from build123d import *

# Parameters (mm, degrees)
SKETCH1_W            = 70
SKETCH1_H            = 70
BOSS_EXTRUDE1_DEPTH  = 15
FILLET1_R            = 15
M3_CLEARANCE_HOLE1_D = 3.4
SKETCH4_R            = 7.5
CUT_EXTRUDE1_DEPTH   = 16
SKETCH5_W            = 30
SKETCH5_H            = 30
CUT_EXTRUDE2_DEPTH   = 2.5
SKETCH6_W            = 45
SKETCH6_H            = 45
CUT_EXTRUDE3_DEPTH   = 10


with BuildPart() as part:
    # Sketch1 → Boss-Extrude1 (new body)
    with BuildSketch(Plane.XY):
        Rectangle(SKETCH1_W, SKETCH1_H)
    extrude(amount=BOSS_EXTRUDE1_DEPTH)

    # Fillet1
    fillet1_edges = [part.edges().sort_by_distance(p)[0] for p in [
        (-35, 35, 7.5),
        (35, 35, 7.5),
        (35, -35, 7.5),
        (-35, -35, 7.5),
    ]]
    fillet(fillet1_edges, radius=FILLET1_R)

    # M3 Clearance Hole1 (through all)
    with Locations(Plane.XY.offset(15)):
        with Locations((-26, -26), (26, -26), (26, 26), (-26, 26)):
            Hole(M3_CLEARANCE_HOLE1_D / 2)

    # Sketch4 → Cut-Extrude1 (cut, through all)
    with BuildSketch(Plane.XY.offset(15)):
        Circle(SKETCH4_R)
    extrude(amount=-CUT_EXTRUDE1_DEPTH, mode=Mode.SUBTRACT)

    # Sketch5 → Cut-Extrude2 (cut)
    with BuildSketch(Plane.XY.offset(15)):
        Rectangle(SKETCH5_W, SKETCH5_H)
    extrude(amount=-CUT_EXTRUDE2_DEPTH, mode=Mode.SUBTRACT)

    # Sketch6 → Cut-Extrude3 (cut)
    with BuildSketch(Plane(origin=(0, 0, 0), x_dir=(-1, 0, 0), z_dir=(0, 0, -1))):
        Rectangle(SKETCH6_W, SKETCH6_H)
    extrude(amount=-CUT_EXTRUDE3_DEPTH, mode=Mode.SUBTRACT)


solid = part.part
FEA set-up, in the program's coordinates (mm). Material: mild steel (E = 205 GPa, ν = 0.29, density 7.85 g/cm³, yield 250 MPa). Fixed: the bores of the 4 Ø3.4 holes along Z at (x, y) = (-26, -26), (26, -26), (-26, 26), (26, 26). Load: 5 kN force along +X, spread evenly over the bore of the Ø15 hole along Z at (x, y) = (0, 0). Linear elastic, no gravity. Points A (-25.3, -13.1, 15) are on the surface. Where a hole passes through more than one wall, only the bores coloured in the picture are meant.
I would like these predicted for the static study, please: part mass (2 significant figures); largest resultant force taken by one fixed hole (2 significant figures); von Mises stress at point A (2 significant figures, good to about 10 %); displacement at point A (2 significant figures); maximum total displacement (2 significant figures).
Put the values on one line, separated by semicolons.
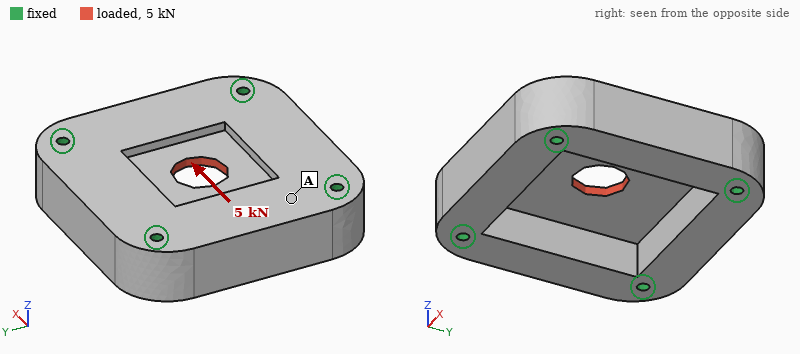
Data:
370 g; 1.3 kN; 10 MPa; 1.4 µm; 4.1 µm
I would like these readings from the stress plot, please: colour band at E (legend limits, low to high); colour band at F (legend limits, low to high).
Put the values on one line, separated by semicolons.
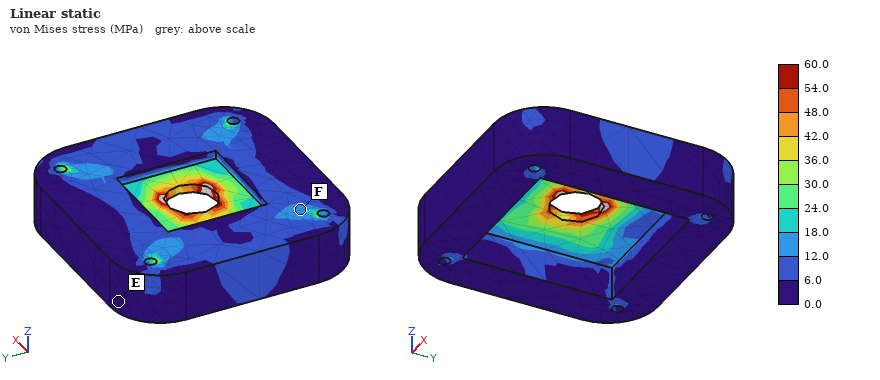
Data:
0.0 to 6.0 MPa; 12.0 to 18.0 MPa
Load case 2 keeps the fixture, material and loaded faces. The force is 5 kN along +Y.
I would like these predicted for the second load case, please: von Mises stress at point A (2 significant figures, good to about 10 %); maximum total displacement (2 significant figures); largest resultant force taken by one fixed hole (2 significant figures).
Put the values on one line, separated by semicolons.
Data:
5.9 MPa; 4.1 µm; 1.3 kN
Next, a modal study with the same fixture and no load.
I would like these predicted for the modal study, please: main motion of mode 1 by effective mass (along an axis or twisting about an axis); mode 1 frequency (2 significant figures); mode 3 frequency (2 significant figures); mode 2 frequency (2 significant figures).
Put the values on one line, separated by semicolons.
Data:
along Z; 14 kHz; 17 kHz; 17 kHz
